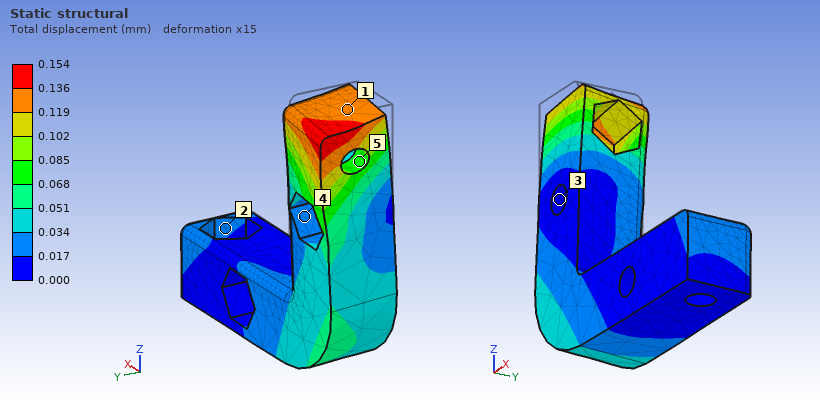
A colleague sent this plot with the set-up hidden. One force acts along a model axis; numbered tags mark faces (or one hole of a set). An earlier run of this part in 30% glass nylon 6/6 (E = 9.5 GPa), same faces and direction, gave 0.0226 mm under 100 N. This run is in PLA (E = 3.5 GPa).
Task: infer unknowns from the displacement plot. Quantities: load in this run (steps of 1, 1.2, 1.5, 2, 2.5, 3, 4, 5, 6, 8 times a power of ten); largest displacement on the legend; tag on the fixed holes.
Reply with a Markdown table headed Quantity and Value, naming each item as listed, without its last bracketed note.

| Quantity | Value |
|---|---|
| load in this run | 250 N |
| largest displacement on the legend | 0.154 mm |
| tag on the fixed holes | 3 |
